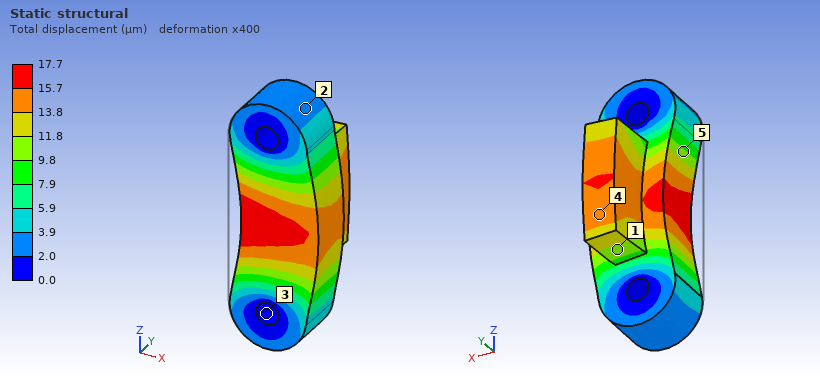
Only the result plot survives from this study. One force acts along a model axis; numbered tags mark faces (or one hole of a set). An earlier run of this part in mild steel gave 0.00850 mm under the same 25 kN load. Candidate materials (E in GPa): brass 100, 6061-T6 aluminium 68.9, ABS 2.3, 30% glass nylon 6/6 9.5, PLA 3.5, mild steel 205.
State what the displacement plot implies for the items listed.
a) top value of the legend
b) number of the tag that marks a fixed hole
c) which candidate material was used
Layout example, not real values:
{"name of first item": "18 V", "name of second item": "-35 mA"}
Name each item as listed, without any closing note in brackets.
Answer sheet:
{"top value of the legend": "17.7 µm", "number of the tag that marks a fixed hole": "3", "which candidate material was used": "brass"}
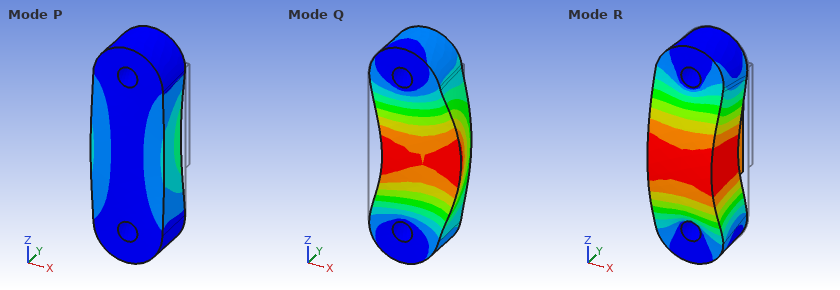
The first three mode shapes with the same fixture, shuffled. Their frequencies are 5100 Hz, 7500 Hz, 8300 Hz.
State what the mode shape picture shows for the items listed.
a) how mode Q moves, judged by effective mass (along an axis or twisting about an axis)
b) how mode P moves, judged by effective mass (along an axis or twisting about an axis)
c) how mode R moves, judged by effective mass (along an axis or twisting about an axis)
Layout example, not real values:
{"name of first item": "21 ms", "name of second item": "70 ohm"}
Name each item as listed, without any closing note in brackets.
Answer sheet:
{"how mode Q moves, judged by effective mass": "along X", "how mode P moves, judged by effective mass": "along X", "how mode R moves, judged by effective mass": "along Y"}
